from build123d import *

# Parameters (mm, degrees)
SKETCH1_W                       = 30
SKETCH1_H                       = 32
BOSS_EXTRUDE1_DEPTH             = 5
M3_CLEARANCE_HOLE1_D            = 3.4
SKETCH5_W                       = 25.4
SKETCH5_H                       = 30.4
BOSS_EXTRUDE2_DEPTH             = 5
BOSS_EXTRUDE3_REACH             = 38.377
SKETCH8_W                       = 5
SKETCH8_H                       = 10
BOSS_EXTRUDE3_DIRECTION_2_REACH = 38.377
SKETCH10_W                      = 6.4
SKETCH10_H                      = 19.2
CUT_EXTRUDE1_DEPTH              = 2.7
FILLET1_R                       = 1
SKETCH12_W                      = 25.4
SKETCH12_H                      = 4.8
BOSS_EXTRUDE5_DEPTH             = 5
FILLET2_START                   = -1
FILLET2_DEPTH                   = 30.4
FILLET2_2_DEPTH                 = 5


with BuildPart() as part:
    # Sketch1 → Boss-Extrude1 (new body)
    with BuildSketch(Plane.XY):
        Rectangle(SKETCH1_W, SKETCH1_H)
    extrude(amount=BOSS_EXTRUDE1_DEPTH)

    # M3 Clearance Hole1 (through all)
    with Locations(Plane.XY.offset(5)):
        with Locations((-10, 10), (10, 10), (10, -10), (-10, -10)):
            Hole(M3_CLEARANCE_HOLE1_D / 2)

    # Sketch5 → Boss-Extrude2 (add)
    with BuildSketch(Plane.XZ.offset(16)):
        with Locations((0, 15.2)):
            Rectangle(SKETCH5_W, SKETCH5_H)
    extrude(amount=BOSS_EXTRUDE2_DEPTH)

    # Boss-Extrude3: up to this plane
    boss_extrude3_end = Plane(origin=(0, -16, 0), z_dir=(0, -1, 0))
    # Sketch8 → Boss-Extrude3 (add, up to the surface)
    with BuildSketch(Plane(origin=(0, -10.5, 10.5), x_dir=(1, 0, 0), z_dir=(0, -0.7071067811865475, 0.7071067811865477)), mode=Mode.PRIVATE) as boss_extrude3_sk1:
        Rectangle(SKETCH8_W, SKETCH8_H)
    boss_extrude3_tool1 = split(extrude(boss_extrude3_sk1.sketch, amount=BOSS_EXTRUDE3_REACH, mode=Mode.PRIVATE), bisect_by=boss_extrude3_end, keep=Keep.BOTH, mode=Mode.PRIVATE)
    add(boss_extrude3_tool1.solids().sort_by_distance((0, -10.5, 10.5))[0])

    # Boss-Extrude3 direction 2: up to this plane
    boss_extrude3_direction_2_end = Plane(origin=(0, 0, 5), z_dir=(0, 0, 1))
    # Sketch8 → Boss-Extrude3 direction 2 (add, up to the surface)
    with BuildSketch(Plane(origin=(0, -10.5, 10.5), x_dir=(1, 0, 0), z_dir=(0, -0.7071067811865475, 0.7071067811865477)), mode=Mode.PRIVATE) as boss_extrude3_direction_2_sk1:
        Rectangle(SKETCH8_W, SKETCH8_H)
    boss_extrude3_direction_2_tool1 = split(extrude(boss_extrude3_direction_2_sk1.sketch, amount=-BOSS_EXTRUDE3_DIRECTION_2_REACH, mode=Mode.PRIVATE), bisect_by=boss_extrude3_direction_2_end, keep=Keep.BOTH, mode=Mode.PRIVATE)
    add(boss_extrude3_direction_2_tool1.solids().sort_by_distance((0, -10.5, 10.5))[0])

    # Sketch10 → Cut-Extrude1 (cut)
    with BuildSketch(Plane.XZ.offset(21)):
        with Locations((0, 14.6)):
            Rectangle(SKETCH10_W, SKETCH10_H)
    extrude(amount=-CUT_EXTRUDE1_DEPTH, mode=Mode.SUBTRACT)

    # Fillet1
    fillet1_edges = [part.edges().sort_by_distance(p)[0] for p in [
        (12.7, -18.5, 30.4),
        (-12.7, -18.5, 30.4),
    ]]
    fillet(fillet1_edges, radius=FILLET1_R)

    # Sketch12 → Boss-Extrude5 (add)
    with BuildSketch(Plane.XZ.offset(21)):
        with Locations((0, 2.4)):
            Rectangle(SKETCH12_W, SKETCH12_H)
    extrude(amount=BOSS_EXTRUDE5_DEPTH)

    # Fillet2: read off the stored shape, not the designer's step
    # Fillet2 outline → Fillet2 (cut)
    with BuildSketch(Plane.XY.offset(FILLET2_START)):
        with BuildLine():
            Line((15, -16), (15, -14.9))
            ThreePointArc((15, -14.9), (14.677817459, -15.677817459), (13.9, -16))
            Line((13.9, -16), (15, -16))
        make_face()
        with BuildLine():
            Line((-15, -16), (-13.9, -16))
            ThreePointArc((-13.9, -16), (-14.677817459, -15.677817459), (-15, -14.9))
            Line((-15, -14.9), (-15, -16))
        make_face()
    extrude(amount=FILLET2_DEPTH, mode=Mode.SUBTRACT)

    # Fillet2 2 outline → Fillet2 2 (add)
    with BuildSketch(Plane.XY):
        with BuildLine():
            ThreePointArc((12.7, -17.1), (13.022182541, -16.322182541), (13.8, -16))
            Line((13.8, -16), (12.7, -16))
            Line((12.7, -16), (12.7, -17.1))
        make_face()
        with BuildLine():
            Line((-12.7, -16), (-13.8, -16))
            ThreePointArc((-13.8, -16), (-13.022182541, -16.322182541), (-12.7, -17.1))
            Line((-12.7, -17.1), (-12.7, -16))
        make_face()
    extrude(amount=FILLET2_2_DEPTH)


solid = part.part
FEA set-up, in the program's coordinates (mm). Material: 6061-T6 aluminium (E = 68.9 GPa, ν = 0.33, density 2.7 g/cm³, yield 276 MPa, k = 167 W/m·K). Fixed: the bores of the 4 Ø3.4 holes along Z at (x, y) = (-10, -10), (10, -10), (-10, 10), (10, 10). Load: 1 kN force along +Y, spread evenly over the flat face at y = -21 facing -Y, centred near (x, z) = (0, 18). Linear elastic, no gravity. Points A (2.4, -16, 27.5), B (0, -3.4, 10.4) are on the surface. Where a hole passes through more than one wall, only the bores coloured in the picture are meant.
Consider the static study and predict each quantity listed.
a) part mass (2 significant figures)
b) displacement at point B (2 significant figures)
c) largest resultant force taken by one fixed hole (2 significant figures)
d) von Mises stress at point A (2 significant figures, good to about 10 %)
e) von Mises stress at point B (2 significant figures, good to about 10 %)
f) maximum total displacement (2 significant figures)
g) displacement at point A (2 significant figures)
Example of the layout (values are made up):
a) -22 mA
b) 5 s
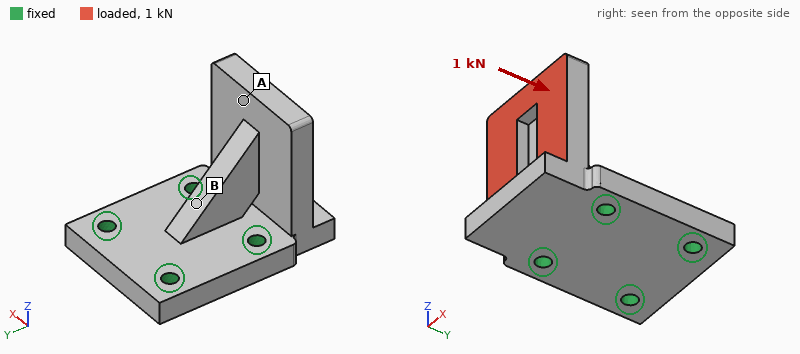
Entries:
a) 26 g
b) 12 µm
c) 390 N
d) 14 MPa
e) 52 MPa
f) 76 µm
g) 58 µm
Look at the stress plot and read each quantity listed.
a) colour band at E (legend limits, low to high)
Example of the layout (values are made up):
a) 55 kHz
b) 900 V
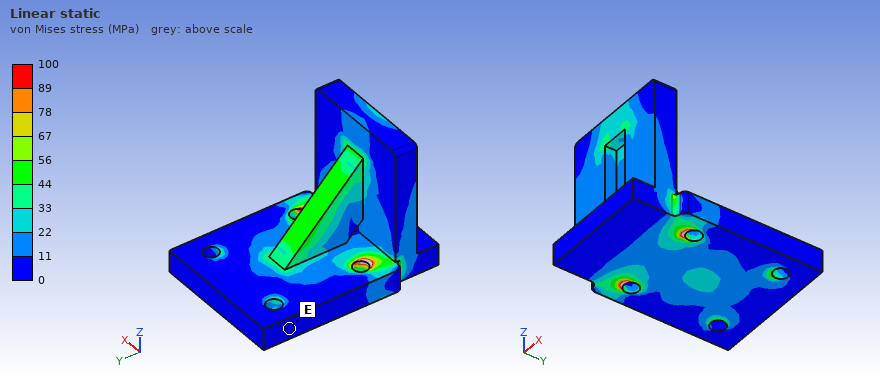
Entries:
a) 0 to 11 MPa
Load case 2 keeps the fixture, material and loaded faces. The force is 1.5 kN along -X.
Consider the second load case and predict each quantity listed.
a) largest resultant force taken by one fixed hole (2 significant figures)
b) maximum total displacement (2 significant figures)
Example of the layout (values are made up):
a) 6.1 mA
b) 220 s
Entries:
a) 1.5 kN
b) 70 µm
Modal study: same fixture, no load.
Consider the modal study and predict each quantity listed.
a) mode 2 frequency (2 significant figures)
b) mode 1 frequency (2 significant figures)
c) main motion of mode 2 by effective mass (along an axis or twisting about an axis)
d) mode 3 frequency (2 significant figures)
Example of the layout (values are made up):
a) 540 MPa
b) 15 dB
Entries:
a) 10 kHz
b) 7500 Hz
c) along X
d) 12 kHz
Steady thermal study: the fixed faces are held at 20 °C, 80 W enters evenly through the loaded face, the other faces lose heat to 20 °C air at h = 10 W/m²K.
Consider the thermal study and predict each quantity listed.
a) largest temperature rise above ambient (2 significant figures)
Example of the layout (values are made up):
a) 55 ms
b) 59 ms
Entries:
a) 73 K
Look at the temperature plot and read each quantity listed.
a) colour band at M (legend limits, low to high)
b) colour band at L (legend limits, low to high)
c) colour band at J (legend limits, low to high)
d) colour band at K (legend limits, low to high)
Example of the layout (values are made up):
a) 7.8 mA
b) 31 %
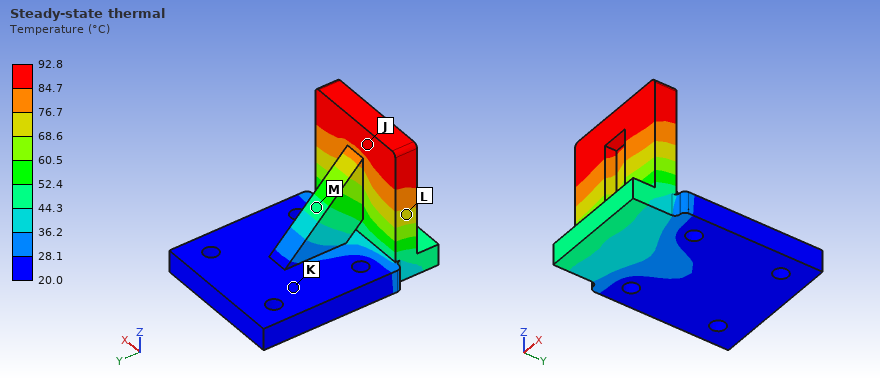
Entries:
a) 44.3 to 52.4 °C
b) 68.6 to 76.7 °C
c) 84.7 to 92.8 °C
d) 20.0 to 28.1 °C
